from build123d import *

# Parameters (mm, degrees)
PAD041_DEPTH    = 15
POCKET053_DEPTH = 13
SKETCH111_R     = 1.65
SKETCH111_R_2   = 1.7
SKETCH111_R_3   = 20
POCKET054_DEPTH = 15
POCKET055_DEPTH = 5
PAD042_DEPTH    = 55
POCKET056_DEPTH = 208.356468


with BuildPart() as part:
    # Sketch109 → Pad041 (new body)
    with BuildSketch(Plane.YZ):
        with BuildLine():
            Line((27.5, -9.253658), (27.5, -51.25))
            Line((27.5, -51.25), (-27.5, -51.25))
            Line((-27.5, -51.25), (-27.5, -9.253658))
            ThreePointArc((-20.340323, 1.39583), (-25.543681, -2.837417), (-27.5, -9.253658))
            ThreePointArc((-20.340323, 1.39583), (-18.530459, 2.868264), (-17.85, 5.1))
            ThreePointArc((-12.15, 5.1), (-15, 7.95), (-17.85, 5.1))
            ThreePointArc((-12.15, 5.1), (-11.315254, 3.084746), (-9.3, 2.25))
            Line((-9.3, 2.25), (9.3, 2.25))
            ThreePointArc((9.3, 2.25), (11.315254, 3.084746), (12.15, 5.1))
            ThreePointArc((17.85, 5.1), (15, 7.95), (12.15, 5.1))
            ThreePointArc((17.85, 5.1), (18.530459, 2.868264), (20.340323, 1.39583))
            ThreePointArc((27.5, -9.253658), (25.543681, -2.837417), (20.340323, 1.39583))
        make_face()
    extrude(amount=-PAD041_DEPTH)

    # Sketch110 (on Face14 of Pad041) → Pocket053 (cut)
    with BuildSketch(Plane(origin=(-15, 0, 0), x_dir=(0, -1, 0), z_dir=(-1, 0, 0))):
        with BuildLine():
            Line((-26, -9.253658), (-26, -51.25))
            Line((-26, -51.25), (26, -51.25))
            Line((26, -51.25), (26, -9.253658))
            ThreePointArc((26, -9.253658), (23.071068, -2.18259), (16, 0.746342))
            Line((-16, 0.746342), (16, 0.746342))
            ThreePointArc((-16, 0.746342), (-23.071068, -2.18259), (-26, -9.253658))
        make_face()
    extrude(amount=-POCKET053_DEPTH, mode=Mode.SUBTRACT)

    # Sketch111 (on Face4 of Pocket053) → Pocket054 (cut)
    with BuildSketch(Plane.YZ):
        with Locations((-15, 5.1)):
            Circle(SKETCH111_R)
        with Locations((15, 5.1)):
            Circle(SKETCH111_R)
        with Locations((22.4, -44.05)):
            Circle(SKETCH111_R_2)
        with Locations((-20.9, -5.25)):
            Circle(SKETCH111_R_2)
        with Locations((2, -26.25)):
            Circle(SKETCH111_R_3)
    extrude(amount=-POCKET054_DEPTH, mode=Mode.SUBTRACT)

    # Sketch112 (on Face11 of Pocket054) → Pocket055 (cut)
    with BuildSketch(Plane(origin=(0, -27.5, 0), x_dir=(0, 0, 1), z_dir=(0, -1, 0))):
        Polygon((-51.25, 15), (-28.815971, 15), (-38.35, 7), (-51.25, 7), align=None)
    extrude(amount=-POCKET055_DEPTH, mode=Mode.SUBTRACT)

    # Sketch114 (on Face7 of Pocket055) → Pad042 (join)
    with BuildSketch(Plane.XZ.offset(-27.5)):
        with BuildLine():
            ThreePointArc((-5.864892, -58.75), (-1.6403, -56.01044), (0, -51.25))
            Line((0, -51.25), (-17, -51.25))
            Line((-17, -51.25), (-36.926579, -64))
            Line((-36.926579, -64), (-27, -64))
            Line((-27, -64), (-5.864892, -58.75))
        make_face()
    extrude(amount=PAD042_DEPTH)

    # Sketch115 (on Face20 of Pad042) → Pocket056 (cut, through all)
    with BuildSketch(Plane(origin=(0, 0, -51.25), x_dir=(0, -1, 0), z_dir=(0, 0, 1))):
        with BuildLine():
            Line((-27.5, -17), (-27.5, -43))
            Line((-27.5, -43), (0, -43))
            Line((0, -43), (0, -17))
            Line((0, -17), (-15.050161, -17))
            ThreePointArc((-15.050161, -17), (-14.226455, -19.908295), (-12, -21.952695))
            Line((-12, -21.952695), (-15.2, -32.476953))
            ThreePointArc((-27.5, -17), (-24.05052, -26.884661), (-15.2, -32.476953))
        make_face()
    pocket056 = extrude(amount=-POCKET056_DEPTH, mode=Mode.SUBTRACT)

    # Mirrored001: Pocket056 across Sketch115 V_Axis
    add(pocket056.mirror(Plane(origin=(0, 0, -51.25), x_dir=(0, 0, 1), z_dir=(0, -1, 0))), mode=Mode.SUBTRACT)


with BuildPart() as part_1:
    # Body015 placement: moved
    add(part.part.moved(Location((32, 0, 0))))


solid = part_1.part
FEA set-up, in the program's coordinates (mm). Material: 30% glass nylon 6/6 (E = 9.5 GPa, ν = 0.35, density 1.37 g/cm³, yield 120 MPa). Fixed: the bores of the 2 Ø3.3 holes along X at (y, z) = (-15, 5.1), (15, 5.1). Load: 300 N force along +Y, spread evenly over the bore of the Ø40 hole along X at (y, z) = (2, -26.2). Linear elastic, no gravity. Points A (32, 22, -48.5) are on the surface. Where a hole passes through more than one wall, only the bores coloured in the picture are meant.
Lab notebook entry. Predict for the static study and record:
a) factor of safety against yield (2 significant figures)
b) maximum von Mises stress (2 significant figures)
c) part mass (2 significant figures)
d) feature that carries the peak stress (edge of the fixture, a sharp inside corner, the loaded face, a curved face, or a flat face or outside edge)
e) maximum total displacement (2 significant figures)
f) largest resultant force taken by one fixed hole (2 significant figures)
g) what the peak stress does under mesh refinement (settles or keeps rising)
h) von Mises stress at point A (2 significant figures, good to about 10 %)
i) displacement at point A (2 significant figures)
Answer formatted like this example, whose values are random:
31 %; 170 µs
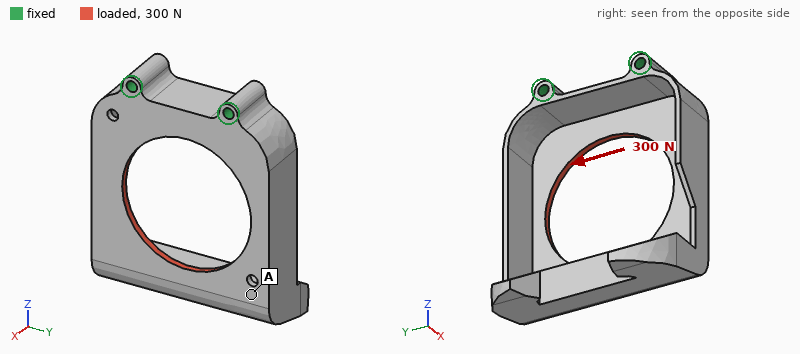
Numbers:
2.6; 46 MPa; 22 g; a curved face; 0.72 mm; 300 N; settles; 5.3 MPa; 0.47 mm
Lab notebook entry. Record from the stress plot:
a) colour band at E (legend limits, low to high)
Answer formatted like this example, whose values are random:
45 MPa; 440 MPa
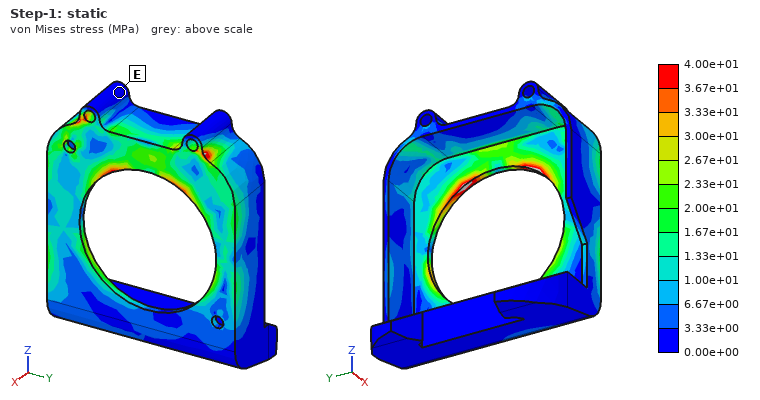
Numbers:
0.00e+00 to 3.33e+00 MPa
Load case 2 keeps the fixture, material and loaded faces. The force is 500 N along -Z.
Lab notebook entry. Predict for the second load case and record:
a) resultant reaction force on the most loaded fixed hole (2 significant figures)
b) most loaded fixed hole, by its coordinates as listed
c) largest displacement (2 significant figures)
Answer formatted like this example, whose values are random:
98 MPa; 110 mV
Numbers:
280 N; (15, 5.1); 0.29 mm
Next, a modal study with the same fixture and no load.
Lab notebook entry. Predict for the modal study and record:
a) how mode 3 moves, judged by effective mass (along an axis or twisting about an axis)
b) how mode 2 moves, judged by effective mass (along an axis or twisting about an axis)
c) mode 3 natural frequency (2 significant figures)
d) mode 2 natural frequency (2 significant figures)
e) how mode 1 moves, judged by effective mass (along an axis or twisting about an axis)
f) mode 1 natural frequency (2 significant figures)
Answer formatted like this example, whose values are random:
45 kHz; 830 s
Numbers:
along Y; along Y; 960 Hz; 440 Hz; along X; 230 Hz
